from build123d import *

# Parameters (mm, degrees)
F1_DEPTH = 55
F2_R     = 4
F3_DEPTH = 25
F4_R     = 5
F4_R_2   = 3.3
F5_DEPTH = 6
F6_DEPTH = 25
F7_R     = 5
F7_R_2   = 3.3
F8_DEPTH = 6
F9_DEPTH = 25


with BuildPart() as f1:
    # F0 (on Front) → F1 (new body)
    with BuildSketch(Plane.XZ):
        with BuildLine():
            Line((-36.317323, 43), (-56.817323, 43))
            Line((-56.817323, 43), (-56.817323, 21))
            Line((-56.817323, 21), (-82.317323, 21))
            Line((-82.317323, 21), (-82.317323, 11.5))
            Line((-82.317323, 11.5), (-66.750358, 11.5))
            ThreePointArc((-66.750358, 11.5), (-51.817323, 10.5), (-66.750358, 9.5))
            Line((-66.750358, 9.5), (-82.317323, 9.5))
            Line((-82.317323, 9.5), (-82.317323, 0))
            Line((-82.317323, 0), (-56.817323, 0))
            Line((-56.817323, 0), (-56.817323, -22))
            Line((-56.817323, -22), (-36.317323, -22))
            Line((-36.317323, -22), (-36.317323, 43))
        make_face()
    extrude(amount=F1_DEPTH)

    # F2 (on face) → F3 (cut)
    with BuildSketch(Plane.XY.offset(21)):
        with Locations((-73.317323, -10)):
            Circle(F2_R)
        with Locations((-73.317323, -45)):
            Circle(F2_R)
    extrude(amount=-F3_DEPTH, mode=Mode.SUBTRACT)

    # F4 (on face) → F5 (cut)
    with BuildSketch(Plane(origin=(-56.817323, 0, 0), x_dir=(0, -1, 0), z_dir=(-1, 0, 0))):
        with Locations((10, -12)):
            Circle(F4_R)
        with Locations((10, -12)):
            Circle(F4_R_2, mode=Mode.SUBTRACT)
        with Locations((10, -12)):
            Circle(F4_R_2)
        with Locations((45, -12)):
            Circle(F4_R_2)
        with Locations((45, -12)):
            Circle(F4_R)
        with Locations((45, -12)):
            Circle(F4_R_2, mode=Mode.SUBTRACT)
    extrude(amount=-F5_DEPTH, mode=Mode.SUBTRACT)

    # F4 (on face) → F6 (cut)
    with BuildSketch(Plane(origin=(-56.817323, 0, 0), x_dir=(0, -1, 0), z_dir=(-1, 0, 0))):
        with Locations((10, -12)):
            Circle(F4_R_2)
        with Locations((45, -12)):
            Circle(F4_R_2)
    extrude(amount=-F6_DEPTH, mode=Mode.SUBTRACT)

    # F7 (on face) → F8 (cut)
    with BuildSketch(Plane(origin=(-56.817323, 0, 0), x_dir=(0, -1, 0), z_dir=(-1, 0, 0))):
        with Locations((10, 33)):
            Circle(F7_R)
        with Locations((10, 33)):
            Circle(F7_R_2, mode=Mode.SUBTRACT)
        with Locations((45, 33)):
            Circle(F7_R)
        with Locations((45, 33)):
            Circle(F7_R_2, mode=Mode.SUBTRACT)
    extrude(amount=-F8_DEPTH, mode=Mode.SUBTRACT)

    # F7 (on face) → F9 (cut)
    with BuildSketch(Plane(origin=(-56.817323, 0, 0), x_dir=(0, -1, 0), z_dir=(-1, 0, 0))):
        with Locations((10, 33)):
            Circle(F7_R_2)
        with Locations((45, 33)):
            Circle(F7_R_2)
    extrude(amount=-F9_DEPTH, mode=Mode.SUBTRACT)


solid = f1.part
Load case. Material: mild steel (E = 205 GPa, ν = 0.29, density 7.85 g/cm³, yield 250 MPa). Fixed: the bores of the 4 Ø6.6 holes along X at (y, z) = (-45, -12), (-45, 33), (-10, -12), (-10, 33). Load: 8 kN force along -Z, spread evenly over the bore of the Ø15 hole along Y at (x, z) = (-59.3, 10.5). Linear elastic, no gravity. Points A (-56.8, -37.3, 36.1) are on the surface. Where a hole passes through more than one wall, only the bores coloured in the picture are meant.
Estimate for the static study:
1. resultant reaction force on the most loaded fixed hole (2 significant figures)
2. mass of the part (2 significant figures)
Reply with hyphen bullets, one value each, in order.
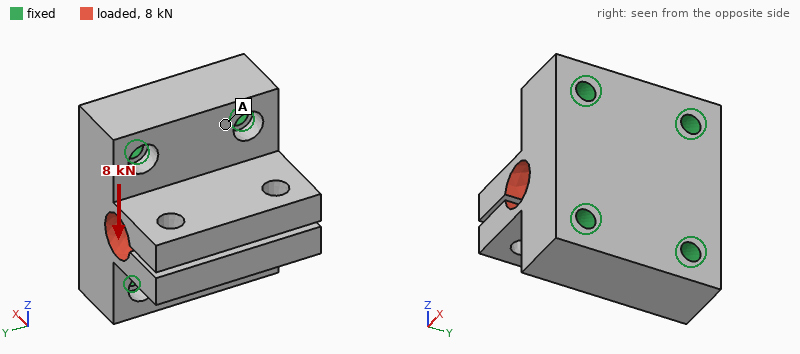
- 2.4 kN
- 670 g
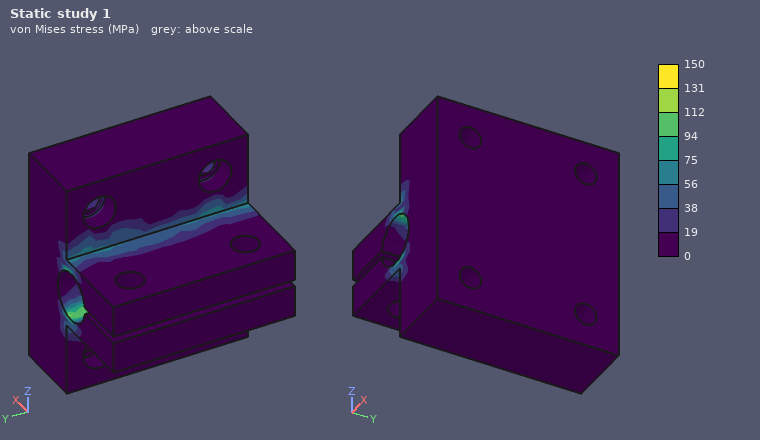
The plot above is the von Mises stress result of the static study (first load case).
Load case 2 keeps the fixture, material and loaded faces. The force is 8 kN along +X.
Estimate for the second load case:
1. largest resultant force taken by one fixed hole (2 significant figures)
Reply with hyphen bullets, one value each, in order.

- 2.0 kN
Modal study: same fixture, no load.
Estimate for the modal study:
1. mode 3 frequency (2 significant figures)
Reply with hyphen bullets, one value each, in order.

- 7100 Hz
